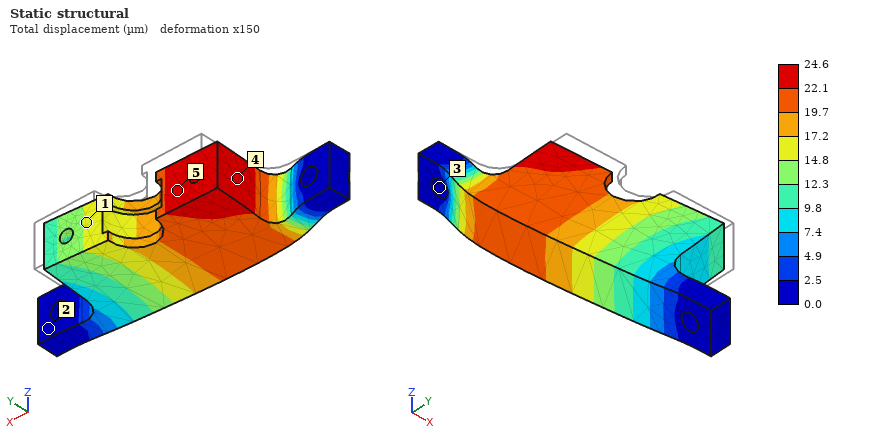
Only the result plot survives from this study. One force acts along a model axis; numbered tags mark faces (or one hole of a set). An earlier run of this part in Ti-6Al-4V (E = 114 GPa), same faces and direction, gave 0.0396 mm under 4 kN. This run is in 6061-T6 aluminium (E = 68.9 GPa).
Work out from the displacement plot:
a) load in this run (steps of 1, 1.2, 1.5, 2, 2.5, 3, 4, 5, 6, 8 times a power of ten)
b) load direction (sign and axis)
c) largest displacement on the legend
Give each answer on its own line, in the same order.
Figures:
1.5 kN
-Y
24.6 µm
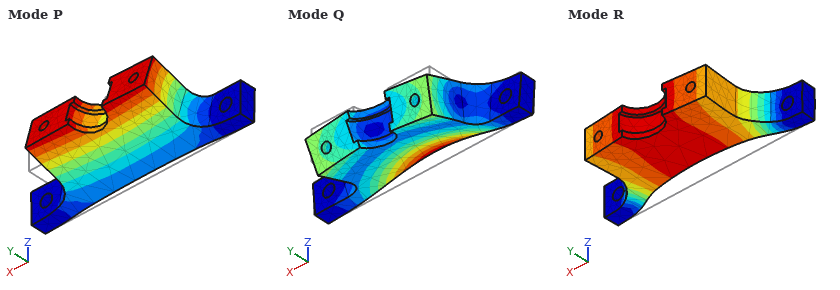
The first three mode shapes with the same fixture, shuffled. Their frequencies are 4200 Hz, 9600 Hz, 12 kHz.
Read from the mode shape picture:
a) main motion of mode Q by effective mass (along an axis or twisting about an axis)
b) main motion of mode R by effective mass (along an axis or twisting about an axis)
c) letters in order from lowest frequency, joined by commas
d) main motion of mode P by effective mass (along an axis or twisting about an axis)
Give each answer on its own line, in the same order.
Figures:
along Z
along Y
P, R, Q
along Z
